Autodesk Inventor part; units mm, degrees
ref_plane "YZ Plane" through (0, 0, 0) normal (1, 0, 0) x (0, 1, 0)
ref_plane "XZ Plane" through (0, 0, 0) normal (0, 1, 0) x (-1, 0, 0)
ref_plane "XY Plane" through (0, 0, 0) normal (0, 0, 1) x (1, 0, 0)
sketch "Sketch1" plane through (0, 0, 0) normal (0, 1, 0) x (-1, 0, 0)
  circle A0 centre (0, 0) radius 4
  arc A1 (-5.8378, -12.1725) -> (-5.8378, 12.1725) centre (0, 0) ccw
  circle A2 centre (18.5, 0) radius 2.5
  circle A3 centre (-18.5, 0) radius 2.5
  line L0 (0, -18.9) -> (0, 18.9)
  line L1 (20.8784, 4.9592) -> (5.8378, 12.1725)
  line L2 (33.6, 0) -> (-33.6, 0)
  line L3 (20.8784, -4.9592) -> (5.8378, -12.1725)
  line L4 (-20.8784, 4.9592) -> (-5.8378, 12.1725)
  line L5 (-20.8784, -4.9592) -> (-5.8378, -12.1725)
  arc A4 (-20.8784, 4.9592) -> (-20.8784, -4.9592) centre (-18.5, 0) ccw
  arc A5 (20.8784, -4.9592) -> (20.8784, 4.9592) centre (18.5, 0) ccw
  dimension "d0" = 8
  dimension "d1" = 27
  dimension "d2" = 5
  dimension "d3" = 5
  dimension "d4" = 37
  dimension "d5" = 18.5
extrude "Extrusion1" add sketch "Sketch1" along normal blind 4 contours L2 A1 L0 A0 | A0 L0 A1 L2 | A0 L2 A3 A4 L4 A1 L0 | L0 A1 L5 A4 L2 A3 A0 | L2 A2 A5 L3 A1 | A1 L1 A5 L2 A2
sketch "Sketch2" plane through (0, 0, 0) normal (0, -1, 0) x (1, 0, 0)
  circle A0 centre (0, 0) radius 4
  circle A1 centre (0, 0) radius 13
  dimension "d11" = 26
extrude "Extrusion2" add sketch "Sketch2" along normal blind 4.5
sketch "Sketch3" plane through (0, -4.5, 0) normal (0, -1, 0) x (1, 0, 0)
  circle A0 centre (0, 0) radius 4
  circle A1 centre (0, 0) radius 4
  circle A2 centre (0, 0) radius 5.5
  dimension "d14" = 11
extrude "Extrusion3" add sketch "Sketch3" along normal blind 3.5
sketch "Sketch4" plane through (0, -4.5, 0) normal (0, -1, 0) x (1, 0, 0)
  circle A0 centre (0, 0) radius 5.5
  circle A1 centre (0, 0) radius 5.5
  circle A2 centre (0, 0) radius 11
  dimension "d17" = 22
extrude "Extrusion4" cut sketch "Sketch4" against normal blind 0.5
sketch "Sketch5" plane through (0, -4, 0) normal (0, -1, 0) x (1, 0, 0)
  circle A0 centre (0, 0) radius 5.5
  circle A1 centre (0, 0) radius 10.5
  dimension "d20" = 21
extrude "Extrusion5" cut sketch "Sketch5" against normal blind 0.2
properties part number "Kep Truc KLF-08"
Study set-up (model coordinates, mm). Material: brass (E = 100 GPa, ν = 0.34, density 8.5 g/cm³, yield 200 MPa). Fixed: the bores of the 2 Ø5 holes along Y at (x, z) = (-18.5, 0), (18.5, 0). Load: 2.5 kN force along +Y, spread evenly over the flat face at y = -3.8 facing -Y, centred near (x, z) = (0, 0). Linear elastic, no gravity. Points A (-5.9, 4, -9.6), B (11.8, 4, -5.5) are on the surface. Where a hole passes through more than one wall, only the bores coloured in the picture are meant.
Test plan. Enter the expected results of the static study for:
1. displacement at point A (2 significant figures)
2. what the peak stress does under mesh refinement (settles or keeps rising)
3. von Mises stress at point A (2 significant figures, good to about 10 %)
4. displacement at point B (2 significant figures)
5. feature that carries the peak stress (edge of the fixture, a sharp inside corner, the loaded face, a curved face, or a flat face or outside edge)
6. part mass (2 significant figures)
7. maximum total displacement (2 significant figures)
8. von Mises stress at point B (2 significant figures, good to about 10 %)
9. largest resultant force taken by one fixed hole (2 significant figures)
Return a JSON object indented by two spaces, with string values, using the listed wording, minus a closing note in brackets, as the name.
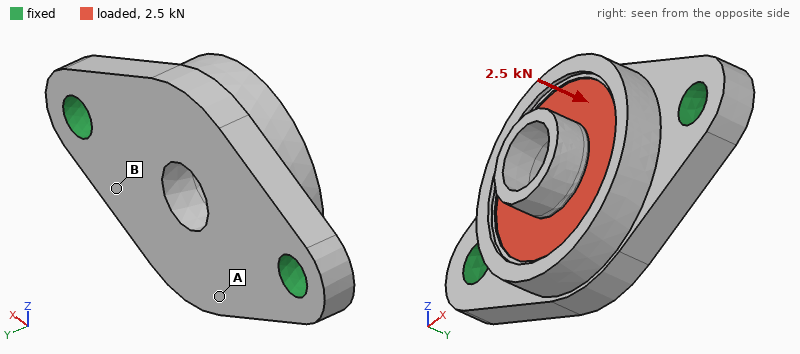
{
  "displacement at point A": "18 µm",
  "what the peak stress does under mesh refinement": "keeps rising",
  "von Mises stress at point A": "27 MPa",
  "displacement at point B": "11 µm",
  "feature that carries the peak stress": "edge of the fixture",
  "part mass": "44 g",
  "maximum total displacement": "21 µm",
  "von Mises stress at point B": "17 MPa",
  "largest resultant force taken by one fixed hole": "1.5 kN"
}
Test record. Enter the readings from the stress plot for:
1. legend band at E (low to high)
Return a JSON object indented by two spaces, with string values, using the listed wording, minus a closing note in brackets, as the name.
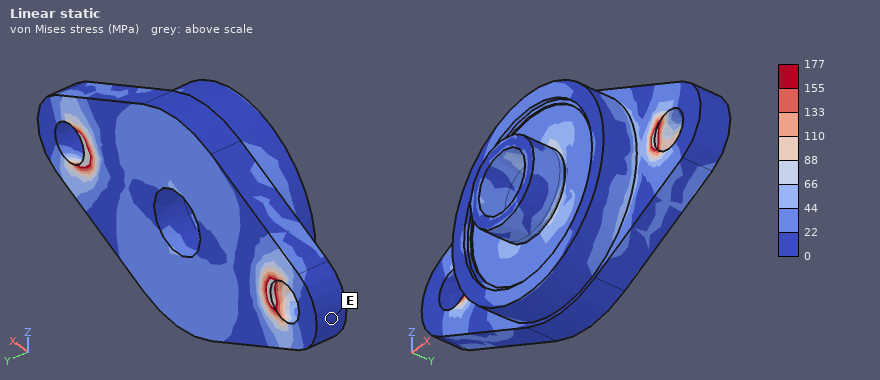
{
  "legend band at E": "0 to 22 MPa"
}
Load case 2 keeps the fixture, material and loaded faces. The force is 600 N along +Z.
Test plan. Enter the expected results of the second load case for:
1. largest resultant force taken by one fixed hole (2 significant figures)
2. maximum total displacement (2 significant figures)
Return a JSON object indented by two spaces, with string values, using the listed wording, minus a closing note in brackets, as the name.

{
  "largest resultant force taken by one fixed hole": "300 N",
  "maximum total displacement": "13 µm"
}
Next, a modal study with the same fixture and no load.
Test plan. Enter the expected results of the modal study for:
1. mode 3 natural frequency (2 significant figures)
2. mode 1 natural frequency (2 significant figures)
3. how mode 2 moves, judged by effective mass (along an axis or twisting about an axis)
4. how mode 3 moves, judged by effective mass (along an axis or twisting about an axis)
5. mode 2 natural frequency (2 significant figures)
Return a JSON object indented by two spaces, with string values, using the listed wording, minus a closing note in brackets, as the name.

{
  "mode 3 natural frequency": "18 kHz",
  "mode 1 natural frequency": "7000 Hz",
  "how mode 2 moves, judged by effective mass": "along Y",
  "how mode 3 moves, judged by effective mass": "along Z",
  "mode 2 natural frequency": "10 kHz"
}
